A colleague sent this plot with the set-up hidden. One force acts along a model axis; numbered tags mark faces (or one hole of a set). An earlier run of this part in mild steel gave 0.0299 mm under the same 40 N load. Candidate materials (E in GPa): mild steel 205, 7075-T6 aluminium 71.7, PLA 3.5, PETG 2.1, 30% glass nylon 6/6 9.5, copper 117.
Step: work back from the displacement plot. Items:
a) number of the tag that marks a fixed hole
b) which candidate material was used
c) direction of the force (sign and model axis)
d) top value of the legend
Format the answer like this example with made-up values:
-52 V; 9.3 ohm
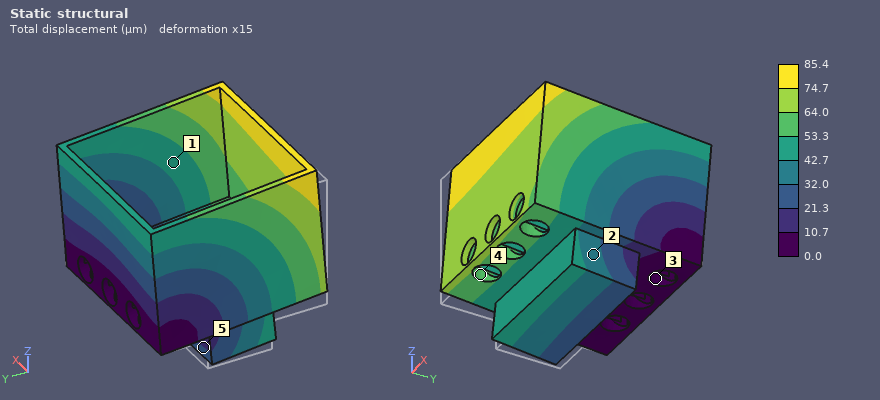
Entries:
3; 7075-T6 aluminium; +Z; 85.4 µm
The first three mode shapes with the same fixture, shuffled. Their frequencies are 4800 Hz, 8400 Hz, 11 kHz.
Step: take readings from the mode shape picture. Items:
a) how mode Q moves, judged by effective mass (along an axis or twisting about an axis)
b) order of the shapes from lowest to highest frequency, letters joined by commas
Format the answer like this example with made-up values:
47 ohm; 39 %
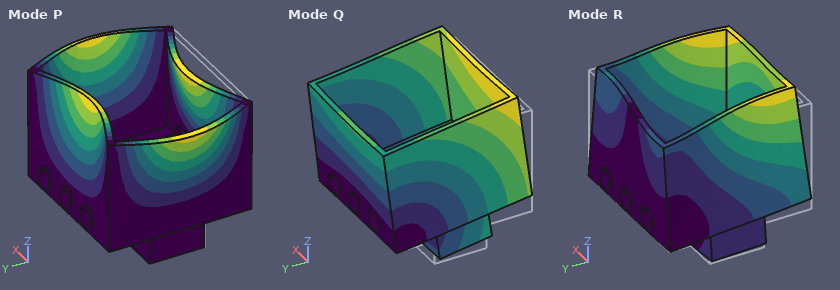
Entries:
along Z; Q, R, P
